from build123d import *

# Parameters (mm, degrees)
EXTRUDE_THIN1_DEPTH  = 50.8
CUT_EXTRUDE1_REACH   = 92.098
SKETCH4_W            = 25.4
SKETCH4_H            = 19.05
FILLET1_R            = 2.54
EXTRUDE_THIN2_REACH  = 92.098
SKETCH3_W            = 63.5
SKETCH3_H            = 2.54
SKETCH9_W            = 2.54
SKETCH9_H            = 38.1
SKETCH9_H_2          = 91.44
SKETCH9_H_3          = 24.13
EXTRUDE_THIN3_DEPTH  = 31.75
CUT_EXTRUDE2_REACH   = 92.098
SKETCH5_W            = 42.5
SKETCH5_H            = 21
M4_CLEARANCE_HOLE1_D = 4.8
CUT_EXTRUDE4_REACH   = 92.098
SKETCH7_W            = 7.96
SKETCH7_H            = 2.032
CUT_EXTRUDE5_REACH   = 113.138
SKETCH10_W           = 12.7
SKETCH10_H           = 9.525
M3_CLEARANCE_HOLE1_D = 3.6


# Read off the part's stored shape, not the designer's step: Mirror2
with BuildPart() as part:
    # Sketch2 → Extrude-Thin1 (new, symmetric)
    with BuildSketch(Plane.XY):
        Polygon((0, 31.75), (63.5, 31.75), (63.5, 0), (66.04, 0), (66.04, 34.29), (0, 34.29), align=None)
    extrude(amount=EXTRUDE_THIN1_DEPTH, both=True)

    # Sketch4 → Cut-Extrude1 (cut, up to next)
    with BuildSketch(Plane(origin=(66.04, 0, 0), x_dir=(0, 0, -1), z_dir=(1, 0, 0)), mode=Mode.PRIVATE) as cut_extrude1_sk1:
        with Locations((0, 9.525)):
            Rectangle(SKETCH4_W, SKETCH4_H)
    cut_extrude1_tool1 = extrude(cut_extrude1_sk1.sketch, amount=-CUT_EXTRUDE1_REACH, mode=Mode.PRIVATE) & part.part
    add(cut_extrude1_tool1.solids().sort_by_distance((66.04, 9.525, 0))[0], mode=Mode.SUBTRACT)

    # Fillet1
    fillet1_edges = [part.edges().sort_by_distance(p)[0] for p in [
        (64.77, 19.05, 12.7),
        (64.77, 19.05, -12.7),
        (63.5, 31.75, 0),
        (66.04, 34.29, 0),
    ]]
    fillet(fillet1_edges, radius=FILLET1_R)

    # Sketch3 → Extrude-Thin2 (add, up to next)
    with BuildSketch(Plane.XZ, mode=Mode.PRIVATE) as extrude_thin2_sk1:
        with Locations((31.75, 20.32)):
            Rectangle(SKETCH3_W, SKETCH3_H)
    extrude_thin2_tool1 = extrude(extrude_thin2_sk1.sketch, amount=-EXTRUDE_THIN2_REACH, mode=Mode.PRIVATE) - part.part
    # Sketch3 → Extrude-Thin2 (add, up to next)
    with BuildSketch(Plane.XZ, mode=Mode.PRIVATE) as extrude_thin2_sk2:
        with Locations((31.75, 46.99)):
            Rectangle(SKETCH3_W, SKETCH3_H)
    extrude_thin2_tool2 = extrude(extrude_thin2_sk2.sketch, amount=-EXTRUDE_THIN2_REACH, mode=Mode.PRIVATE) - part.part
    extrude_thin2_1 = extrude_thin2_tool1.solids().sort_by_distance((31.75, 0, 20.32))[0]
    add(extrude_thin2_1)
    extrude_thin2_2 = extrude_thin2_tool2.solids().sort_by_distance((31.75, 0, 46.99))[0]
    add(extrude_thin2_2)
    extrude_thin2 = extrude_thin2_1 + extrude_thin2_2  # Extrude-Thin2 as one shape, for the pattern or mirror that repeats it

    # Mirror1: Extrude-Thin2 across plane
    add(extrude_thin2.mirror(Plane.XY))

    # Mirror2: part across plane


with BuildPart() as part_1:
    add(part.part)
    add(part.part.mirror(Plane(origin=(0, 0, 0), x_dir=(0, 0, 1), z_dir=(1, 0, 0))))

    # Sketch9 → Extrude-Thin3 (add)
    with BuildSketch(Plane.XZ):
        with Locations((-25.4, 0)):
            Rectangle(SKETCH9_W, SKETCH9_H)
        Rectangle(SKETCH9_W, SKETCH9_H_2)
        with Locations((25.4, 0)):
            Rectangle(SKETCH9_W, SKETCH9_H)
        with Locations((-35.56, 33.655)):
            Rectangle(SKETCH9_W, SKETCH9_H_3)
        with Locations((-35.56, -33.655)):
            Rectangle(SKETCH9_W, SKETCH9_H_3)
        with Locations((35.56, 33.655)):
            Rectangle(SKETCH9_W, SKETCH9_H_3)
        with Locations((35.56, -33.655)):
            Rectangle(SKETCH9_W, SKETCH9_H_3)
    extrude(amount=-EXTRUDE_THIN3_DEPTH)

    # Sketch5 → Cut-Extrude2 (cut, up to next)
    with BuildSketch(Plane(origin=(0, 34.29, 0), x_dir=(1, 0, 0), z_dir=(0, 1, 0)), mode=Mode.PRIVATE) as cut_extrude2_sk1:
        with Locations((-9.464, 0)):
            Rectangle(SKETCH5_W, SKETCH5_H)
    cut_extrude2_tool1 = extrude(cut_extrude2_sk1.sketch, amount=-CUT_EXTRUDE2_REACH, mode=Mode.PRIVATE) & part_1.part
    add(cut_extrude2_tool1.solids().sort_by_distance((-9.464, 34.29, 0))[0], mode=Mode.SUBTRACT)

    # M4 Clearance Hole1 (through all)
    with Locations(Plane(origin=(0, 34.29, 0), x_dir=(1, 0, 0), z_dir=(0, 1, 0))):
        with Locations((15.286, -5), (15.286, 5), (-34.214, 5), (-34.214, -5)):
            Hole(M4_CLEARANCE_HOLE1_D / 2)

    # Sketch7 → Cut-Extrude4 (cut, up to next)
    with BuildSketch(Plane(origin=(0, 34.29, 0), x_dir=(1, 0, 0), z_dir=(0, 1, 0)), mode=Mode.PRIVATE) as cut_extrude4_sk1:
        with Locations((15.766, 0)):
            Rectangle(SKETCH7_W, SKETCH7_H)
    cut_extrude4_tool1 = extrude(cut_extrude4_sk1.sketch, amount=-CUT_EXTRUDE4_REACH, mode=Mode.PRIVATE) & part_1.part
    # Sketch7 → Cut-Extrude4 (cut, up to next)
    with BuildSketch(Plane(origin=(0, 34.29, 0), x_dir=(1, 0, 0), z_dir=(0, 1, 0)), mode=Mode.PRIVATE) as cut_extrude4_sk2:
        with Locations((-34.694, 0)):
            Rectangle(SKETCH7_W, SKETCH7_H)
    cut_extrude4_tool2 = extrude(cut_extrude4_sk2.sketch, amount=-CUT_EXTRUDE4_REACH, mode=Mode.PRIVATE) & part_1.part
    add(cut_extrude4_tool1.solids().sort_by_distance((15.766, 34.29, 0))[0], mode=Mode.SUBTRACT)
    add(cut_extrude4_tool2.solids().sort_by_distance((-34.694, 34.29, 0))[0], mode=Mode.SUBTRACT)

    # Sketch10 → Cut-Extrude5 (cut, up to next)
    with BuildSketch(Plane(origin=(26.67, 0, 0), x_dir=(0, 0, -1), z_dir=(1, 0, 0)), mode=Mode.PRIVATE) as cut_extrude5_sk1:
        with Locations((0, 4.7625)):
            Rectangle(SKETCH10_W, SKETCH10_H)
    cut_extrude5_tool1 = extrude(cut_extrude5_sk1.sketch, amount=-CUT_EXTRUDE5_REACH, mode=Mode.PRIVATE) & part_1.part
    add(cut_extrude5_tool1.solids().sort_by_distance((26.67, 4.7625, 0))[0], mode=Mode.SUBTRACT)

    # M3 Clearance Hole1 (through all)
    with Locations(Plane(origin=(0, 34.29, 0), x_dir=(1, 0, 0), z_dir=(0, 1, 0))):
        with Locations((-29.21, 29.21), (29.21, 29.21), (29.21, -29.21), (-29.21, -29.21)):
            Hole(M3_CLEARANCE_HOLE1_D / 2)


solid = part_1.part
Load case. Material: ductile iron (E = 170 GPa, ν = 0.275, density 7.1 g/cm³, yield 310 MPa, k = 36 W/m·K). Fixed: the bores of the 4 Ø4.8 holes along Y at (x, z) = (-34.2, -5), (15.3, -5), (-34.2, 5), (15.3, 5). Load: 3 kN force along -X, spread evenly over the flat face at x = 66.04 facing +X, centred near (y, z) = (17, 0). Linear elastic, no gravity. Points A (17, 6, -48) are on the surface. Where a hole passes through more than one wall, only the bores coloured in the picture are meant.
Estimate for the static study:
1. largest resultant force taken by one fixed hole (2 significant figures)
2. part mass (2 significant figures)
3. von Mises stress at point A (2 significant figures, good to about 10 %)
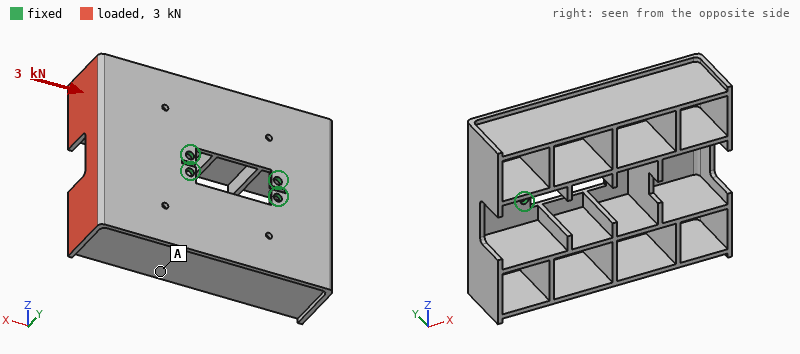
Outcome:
1.0 kN
740 g
6.7 MPa
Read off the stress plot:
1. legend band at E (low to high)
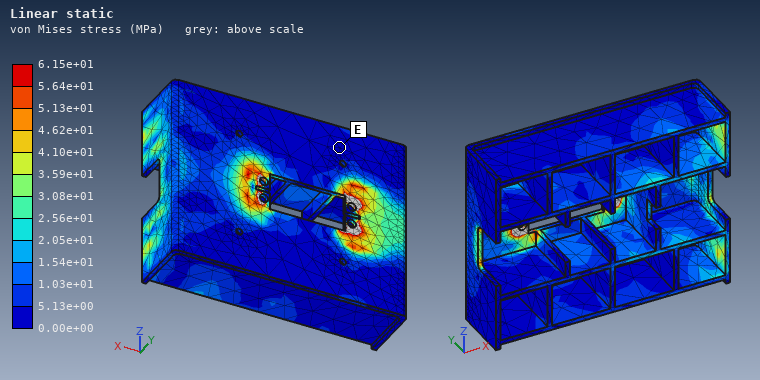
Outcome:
0.00e+00 to 5.13e+00 MPa
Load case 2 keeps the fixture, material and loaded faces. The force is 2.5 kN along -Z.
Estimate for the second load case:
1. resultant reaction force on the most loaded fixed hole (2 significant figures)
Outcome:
3.0 kN
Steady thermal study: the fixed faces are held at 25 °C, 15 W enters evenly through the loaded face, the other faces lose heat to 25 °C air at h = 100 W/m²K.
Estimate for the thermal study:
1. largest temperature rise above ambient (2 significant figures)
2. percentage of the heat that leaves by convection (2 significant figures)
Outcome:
16 K
98 %
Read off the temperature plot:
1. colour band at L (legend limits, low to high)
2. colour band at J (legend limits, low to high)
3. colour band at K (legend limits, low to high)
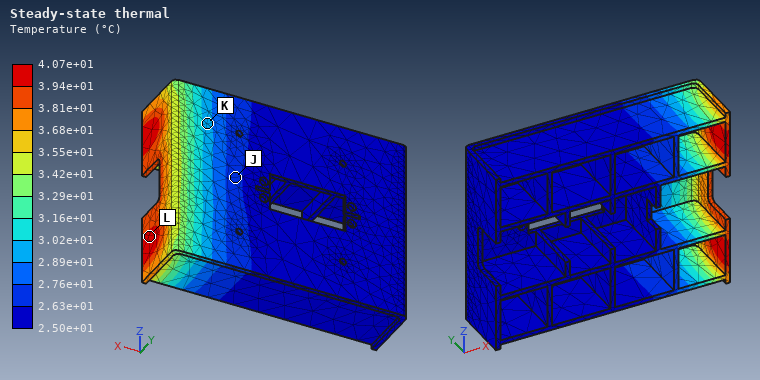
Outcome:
3.94e+01 to 4.07e+01 °C
2.63e+01 to 2.76e+01 °C
2.89e+01 to 3.02e+01 °C
